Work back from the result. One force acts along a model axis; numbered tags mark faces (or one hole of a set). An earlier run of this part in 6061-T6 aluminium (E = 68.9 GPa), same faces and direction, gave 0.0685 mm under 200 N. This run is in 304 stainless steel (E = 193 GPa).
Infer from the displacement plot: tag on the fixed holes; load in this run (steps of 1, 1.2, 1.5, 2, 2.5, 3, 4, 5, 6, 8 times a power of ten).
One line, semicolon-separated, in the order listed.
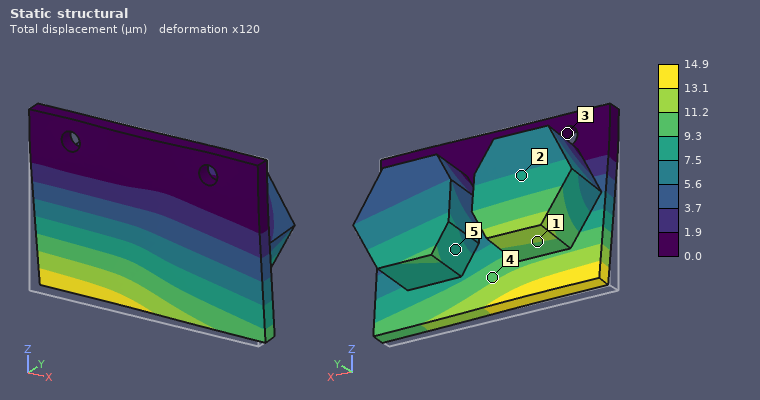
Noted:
3; 120 N
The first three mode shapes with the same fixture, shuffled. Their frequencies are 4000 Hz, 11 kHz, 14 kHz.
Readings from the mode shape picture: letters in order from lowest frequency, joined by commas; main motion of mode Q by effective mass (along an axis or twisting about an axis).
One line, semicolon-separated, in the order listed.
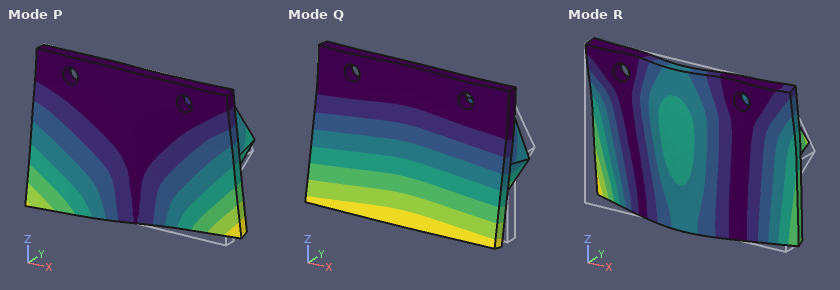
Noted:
Q, P, R; along Y
